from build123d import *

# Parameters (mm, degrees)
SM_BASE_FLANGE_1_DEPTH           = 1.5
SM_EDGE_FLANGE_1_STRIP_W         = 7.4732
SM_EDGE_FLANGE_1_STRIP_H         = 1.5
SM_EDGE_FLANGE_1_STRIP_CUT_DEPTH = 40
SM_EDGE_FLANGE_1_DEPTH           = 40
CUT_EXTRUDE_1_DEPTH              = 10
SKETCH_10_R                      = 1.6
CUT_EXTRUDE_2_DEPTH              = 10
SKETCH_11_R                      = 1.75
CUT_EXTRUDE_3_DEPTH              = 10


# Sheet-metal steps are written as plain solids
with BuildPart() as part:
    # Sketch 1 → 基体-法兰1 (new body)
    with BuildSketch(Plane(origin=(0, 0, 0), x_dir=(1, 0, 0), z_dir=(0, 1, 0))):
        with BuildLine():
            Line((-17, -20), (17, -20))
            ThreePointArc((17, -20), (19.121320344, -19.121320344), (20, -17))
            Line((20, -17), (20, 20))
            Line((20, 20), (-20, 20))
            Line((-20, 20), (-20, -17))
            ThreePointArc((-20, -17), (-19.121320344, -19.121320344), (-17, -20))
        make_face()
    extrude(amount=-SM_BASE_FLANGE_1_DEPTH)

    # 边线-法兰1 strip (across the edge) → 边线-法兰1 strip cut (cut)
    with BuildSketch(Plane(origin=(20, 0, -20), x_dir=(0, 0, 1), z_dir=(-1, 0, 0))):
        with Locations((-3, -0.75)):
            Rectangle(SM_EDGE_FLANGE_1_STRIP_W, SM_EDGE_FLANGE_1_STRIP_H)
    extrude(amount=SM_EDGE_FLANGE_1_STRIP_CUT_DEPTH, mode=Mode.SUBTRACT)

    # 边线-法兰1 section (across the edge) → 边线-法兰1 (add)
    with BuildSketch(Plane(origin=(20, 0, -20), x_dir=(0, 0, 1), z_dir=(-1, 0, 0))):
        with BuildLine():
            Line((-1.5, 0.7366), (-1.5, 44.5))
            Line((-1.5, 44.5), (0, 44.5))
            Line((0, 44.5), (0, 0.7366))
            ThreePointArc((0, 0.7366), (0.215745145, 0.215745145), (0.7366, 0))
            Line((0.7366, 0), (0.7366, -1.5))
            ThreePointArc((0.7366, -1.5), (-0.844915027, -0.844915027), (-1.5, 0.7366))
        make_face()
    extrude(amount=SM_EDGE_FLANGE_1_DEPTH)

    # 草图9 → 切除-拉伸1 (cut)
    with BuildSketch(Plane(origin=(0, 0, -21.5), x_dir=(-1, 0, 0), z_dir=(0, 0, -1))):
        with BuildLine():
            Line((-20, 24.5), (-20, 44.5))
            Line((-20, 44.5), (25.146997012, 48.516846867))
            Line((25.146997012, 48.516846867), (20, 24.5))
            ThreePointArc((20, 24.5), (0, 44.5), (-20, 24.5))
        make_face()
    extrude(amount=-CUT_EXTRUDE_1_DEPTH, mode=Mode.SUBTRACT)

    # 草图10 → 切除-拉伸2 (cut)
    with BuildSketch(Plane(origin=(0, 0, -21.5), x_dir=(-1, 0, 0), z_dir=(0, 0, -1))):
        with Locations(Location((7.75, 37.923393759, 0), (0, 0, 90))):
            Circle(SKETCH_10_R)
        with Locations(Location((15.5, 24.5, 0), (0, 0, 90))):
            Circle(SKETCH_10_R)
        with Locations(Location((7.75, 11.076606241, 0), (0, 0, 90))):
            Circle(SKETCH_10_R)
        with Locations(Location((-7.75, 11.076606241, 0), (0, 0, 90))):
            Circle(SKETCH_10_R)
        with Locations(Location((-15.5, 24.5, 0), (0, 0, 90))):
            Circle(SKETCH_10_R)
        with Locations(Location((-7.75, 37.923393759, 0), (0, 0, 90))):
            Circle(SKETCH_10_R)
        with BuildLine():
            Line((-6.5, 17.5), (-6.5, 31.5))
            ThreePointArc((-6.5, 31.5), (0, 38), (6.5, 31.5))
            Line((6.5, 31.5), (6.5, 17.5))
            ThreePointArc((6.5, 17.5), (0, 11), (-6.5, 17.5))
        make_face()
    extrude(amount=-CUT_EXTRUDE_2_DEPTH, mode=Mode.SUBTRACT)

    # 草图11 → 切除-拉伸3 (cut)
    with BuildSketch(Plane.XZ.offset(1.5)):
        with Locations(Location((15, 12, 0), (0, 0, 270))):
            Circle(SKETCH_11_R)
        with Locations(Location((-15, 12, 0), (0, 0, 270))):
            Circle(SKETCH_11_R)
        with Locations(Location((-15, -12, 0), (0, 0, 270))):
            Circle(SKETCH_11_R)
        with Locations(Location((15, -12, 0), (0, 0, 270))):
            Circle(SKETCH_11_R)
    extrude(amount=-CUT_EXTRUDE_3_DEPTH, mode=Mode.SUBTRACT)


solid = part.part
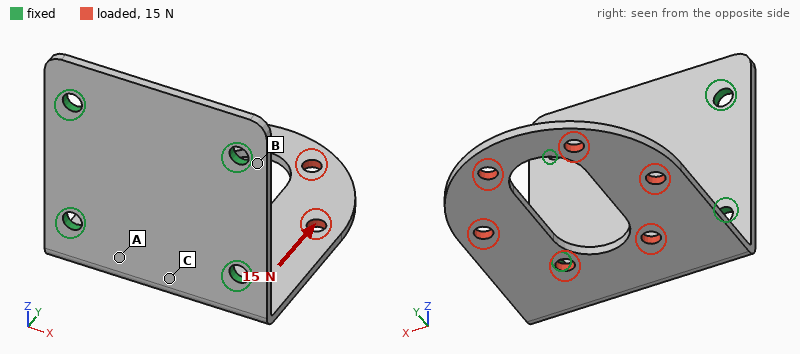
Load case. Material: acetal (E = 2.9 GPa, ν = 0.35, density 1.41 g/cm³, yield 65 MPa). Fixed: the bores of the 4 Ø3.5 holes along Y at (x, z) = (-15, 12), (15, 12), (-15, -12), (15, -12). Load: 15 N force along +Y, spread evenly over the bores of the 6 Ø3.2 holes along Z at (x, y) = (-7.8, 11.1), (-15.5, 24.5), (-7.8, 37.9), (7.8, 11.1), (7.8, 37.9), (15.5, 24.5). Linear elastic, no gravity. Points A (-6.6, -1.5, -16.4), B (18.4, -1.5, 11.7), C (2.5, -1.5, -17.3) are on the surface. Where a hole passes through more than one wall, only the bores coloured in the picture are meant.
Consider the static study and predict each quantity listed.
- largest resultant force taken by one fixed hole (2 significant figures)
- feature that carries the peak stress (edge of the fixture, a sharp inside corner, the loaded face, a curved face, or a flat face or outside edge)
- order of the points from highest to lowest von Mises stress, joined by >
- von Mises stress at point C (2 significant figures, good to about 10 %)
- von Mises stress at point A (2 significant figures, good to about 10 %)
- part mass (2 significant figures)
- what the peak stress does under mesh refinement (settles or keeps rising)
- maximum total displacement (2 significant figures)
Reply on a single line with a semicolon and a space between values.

7.9 N; edge of the fixture; A > C > B; 2.0 MPa; 2.7 MPa; 6.0 g; keeps rising; 0.72 mm
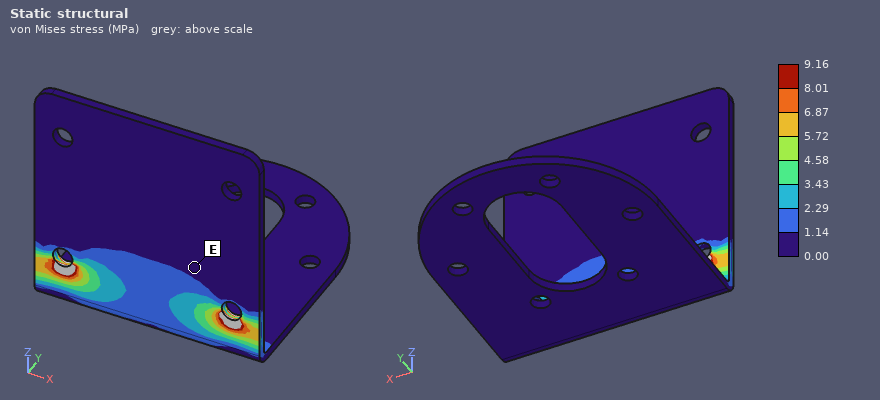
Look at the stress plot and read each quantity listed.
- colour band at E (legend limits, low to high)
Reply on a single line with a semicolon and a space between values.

0.00 to 1.14 MPa
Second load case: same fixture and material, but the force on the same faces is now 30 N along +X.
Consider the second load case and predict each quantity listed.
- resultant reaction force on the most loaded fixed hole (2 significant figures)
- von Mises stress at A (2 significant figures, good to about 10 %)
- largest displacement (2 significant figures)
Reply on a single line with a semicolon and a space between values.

30 N; 5.7 MPa; 0.87 mm
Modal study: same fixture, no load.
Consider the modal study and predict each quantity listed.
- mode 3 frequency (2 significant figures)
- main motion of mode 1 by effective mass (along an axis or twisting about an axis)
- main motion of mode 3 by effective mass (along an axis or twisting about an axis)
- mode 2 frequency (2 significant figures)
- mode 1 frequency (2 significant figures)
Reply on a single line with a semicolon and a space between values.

830 Hz; along Z; along X; 450 Hz; 170 Hz
